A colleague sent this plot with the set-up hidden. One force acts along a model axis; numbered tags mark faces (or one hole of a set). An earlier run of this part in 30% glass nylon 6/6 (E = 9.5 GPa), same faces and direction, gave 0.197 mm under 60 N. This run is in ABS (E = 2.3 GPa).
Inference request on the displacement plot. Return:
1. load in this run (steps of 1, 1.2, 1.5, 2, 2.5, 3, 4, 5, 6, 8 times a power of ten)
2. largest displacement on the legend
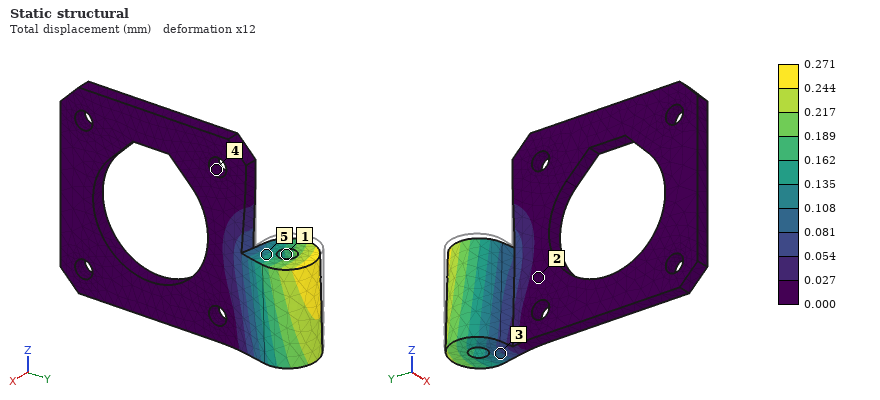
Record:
20 N
0.271 mm
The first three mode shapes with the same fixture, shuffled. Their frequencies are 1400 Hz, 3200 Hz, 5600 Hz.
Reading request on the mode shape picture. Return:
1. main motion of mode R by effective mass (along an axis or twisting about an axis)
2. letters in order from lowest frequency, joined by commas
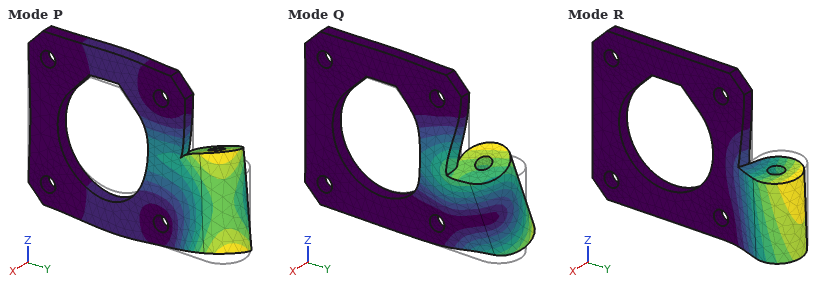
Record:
along X
R, Q, P
